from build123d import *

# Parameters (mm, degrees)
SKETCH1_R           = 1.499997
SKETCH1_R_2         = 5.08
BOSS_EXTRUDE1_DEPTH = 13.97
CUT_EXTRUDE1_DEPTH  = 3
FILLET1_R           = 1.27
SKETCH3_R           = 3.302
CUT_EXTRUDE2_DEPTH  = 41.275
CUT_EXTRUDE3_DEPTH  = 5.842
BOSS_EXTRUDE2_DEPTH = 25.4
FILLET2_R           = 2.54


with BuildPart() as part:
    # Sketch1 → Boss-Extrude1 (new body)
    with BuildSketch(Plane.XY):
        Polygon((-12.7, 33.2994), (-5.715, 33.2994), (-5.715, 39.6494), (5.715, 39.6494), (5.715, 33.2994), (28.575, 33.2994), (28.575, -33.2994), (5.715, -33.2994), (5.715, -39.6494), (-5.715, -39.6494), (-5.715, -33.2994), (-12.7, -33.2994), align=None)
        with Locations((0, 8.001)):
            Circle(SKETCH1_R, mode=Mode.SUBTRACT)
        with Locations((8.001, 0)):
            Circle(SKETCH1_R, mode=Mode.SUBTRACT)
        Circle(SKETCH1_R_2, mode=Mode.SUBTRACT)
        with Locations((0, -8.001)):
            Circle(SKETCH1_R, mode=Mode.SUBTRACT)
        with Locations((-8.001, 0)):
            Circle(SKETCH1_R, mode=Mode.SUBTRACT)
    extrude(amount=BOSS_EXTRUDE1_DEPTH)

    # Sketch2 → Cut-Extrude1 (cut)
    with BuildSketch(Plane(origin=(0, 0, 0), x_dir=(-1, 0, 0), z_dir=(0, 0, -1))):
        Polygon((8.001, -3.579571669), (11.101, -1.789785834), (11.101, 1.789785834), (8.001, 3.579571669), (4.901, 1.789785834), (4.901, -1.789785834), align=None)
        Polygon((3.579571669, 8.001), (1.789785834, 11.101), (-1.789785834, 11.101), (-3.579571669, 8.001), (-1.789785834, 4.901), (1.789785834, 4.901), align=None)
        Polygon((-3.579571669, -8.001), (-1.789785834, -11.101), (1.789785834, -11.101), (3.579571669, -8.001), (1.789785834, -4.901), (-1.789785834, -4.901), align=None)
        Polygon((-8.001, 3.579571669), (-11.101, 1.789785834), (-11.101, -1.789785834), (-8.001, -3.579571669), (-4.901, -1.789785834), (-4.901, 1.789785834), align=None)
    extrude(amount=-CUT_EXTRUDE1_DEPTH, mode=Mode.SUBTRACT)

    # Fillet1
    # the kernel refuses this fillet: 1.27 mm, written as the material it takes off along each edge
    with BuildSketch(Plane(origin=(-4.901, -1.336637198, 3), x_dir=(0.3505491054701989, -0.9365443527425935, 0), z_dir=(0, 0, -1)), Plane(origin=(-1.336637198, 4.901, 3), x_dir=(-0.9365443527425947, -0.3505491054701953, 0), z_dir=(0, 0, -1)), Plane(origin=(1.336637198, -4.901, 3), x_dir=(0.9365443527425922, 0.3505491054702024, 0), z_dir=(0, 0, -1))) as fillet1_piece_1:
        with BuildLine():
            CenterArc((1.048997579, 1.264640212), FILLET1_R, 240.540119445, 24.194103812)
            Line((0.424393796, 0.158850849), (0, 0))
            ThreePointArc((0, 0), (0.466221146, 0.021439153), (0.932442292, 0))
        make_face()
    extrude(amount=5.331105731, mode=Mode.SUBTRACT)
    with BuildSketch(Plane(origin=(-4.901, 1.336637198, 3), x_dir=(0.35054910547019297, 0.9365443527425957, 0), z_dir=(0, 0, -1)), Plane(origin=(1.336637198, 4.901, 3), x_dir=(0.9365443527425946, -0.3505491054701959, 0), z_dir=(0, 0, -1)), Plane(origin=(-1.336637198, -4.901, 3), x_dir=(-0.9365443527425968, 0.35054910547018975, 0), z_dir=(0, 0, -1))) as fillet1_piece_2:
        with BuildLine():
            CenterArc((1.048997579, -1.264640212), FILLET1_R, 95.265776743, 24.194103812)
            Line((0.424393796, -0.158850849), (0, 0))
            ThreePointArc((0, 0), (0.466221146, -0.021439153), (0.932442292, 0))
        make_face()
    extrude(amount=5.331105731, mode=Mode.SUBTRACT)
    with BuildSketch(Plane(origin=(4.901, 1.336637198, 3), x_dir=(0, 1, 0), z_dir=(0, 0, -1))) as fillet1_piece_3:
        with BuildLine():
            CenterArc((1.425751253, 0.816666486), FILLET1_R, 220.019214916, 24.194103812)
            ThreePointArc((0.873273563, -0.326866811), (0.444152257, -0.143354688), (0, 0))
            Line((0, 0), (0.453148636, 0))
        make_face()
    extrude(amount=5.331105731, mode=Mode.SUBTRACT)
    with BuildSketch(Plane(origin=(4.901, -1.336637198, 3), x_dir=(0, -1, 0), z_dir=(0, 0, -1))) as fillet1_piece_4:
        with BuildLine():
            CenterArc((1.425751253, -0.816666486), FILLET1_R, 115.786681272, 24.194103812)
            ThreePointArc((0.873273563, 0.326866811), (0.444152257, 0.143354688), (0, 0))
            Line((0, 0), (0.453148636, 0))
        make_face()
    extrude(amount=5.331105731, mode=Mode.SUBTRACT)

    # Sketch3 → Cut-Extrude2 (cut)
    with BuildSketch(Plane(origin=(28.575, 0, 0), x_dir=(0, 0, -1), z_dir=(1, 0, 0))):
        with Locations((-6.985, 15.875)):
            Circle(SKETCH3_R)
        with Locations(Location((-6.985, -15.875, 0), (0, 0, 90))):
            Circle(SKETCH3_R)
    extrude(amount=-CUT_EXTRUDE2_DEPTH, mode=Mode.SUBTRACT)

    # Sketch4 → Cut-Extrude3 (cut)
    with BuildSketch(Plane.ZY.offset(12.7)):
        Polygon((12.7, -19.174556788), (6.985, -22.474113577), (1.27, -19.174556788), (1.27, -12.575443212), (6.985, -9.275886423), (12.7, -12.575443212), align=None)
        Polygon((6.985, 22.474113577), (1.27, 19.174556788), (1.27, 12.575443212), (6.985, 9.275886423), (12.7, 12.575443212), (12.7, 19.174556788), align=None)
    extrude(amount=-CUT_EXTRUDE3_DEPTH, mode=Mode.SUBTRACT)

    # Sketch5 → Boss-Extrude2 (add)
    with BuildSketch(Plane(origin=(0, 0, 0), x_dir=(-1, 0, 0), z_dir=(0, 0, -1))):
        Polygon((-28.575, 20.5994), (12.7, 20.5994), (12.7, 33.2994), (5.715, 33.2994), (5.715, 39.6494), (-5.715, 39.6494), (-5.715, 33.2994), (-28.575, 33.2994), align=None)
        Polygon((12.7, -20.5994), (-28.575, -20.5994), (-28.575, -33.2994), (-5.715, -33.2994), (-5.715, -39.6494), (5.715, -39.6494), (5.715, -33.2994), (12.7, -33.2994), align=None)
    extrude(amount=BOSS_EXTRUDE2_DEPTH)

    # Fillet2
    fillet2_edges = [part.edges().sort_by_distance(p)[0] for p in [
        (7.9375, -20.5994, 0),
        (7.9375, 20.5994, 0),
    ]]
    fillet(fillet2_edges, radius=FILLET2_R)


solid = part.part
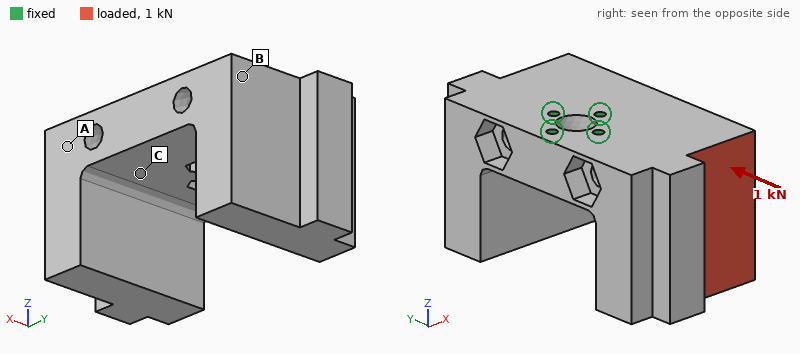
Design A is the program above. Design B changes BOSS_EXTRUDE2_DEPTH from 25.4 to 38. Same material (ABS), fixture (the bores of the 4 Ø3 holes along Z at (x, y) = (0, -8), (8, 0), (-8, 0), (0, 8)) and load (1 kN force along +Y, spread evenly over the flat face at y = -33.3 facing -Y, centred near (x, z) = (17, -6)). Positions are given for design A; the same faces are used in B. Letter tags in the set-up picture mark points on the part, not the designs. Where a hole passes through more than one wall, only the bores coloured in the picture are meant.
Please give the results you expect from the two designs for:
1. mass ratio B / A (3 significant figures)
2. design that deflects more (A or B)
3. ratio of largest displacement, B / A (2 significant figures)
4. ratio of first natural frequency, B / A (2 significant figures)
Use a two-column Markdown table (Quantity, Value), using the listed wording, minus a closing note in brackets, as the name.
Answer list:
| Quantity | Value |
|---|---|
| mass ratio B / A | 1.23 |
| design that deflects more | B |
| ratio of largest displacement, B / A | 1.9 |
| ratio of first natural frequency, B / A | 0.72 |
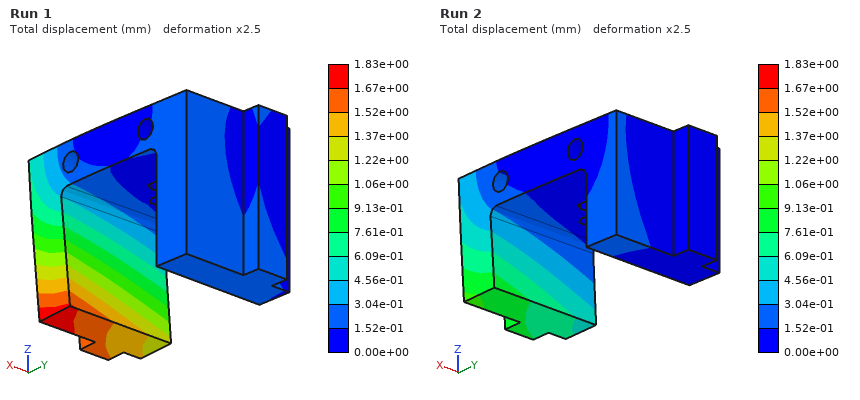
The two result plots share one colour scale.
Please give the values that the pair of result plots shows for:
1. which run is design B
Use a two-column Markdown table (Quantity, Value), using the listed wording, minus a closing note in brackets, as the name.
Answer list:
| Quantity | Value |
|---|---|
| which run is design B | Run 1 |
